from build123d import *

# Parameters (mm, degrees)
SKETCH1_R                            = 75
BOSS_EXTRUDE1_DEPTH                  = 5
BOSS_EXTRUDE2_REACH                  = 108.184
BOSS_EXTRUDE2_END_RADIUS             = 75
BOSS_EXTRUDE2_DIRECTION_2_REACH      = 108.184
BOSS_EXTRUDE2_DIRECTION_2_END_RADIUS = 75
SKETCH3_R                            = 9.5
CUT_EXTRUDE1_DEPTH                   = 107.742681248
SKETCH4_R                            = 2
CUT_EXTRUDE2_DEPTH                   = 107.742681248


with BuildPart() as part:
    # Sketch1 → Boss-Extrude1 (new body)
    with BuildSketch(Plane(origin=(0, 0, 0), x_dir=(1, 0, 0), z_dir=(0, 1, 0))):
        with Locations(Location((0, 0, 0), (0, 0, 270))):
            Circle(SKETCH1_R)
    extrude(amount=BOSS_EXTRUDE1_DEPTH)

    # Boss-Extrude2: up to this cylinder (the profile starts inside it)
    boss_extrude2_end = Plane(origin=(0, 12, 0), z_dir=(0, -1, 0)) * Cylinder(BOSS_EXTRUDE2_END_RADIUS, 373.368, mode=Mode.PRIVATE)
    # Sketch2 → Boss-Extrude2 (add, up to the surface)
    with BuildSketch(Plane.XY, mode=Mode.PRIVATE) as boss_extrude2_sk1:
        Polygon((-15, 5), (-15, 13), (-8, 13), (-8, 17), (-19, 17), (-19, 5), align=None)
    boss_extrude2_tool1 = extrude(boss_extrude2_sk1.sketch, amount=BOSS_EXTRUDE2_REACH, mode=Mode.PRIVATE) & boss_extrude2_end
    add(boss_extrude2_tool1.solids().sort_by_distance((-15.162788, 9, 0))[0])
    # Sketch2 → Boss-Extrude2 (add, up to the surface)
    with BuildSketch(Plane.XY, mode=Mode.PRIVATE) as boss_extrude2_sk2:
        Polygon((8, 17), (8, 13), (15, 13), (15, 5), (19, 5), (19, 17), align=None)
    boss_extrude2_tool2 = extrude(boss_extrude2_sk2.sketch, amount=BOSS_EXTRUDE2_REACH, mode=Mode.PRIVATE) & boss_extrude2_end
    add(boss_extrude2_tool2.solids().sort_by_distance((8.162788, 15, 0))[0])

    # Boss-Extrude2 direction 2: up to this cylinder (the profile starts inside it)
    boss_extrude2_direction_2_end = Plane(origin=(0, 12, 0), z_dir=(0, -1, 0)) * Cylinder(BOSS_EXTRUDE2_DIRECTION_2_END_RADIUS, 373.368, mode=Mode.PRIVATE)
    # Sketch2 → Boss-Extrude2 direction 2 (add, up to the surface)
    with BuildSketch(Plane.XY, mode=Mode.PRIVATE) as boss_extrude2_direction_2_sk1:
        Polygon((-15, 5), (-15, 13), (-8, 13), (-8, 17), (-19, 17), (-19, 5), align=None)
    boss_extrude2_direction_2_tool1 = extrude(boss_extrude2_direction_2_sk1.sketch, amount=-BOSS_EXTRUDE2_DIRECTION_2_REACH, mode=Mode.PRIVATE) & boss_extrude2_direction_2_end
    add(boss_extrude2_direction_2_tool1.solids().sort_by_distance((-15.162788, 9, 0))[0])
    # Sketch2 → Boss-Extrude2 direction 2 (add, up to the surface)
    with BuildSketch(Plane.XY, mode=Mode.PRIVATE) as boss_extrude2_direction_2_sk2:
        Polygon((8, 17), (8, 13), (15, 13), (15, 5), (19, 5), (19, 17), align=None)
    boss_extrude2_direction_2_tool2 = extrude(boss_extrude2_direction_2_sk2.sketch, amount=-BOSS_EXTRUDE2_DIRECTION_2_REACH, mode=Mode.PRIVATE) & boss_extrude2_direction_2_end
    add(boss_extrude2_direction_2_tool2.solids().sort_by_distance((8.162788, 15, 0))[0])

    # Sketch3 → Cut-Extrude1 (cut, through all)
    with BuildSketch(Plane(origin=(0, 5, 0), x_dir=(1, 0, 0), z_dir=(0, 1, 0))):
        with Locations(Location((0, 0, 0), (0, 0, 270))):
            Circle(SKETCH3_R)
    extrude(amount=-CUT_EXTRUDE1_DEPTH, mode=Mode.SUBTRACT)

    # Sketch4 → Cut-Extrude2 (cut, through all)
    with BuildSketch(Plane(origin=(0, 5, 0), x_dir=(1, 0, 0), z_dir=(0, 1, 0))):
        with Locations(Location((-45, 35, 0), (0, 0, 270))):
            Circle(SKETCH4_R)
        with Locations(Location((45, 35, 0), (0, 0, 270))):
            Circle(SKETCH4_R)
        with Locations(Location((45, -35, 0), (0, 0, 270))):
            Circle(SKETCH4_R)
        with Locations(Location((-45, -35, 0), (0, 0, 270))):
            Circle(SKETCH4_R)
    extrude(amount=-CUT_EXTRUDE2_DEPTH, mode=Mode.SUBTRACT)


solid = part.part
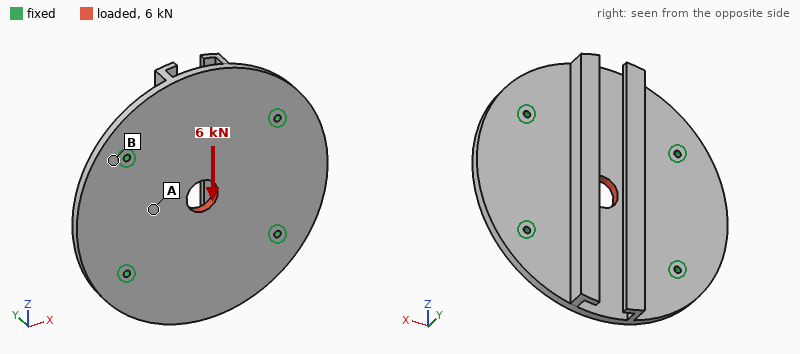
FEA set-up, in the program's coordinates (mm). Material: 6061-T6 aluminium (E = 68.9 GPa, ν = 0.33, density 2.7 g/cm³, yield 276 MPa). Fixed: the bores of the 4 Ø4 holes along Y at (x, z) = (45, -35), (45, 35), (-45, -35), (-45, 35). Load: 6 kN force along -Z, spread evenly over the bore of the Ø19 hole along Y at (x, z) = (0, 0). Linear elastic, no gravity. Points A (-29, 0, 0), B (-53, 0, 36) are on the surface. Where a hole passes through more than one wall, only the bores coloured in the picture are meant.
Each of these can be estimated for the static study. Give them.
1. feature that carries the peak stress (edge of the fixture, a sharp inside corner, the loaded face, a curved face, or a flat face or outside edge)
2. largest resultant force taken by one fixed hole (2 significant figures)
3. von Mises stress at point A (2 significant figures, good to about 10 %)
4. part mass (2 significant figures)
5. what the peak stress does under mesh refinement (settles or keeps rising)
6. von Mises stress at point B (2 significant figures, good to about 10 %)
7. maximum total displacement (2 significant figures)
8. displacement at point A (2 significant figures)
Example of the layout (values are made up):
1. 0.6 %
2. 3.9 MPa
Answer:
1. edge of the fixture
2. 1.5 kN
3. 8.4 MPa
4. 290 g
5. keeps rising
6. 3.4 MPa
7. 13 µm
8. 5.5 µm
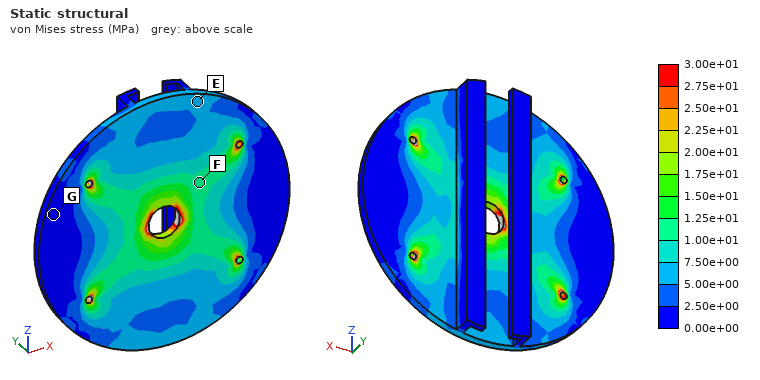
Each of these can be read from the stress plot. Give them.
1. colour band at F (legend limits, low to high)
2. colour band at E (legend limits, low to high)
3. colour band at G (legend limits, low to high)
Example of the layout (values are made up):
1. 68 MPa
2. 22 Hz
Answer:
1. 1.00e+01 to 1.25e+01 MPa
2. 5.00e+00 to 7.50e+00 MPa
3. 0.00e+00 to 2.50e+00 MPa
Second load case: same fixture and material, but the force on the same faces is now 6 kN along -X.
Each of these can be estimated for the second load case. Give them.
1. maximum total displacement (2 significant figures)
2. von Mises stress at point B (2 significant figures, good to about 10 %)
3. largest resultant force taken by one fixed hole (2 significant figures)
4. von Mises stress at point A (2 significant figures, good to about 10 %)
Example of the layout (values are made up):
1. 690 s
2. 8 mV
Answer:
1. 11 µm
2. 8.3 MPa
3. 1.5 kN
4. 8.9 MPa
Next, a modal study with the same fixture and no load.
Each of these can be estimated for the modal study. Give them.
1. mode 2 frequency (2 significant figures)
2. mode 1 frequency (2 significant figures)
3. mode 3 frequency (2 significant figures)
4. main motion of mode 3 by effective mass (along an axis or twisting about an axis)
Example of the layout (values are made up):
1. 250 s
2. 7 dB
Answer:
1. 1800 Hz
2. 1800 Hz
3. 3400 Hz
4. twisting about Z
